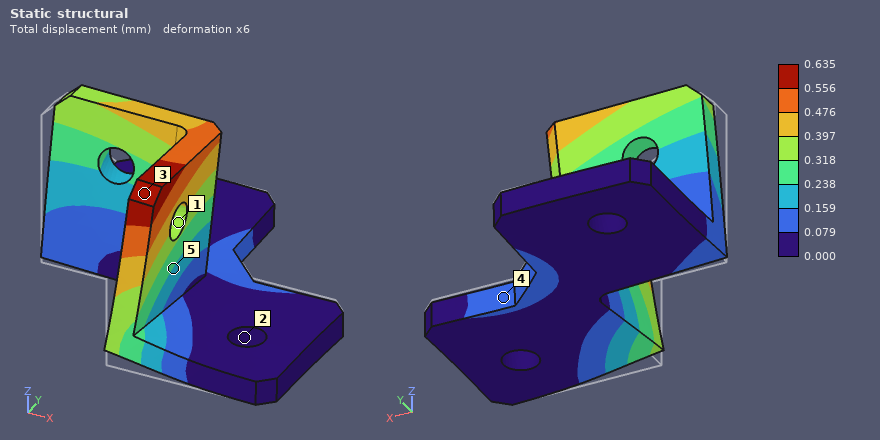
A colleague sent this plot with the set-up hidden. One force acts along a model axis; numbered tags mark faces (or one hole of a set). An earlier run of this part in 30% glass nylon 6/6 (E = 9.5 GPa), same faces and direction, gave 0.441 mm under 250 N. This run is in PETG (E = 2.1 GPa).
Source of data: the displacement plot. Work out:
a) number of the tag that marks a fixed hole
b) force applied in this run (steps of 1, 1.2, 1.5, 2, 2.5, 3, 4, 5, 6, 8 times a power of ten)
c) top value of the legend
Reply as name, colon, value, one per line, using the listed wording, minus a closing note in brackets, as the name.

number of the tag that marks a fixed hole: 2
force applied in this run: 80 N
top value of the legend: 0.635 mm
